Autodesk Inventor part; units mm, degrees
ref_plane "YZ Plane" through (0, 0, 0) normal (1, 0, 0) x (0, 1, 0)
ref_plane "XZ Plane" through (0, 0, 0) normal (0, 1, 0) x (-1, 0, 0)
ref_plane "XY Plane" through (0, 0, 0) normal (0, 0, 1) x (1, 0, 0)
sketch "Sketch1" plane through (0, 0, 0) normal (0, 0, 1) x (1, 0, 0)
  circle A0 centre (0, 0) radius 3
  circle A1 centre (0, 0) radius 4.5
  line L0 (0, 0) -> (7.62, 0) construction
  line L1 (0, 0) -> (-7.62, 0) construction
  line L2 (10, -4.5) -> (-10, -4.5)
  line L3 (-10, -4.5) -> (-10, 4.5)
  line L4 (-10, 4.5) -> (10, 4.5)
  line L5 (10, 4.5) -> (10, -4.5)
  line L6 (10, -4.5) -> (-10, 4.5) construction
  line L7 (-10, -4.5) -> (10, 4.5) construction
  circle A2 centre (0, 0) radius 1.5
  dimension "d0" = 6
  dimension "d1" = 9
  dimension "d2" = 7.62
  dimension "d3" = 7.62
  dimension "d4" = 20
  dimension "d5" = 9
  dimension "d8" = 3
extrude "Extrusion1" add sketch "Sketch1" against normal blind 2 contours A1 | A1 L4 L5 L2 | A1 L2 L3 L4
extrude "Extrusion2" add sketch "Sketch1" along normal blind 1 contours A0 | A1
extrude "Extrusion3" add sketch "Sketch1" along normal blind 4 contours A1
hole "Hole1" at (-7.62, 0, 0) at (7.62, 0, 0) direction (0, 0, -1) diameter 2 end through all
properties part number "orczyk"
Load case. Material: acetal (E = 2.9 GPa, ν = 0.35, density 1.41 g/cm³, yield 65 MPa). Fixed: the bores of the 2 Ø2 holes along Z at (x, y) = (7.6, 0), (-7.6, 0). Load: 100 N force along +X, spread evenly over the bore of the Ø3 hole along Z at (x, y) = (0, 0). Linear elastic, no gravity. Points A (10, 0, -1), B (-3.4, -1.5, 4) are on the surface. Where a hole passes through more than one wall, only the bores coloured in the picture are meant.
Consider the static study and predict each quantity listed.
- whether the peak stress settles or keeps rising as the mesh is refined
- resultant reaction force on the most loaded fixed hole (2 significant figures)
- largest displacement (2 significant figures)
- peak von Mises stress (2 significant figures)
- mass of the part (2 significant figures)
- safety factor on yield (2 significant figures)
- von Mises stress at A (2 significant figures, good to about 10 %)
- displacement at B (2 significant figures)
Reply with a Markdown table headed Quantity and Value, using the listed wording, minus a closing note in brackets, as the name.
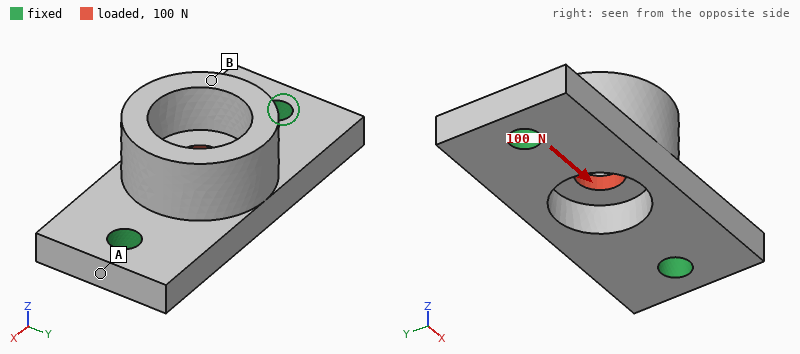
| Quantity | Value |
|---|---|
| whether the peak stress settles or keeps rising as the mesh is refined | settles |
| resultant reaction force on the most loaded fixed hole | 51 N |
| largest displacement | 18 µm |
| peak von Mises stress | 18 MPa |
| mass of the part | 0.64 g |
| safety factor on yield | 3.5 |
| von Mises stress at A | 3.3 MPa |
| displacement at B | 12 µm |
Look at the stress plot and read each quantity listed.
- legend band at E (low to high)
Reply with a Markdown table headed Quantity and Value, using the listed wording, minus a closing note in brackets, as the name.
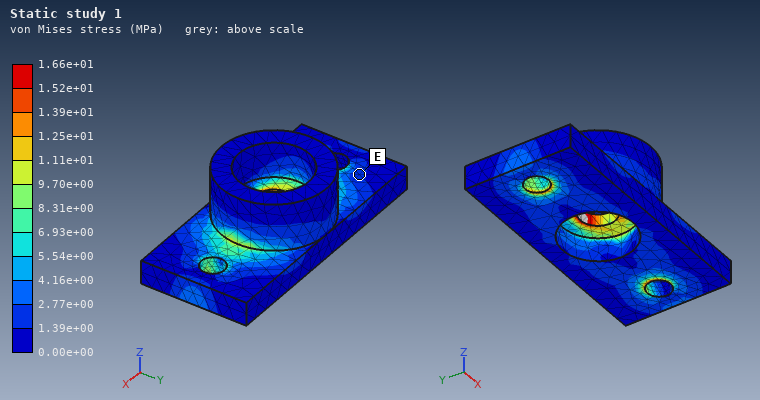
| Quantity | Value |
|---|---|
| legend band at E | 1.39e+00 to 2.77e+00 MPa |
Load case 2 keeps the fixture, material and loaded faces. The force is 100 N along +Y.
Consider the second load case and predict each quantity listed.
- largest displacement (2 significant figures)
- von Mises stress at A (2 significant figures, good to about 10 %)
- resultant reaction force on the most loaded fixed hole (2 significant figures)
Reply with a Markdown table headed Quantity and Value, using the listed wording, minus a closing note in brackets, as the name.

| Quantity | Value |
|---|---|
| largest displacement | 96 µm |
| von Mises stress at A | 4.7 MPa |
| resultant reaction force on the most loaded fixed hole | 50 N |
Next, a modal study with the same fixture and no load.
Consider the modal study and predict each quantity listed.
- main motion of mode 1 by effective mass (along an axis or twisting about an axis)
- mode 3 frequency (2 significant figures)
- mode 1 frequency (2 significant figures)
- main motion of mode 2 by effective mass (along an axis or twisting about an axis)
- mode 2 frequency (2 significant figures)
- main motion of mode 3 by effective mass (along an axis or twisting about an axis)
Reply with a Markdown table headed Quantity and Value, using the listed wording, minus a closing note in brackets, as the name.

| Quantity | Value |
|---|---|
| main motion of mode 1 by effective mass | along Y |
| mode 3 frequency | 18 kHz |
| mode 1 frequency | 7500 Hz |
| main motion of mode 2 by effective mass | along Z |
| mode 2 frequency | 11 kHz |
| main motion of mode 3 by effective mass | along X |
